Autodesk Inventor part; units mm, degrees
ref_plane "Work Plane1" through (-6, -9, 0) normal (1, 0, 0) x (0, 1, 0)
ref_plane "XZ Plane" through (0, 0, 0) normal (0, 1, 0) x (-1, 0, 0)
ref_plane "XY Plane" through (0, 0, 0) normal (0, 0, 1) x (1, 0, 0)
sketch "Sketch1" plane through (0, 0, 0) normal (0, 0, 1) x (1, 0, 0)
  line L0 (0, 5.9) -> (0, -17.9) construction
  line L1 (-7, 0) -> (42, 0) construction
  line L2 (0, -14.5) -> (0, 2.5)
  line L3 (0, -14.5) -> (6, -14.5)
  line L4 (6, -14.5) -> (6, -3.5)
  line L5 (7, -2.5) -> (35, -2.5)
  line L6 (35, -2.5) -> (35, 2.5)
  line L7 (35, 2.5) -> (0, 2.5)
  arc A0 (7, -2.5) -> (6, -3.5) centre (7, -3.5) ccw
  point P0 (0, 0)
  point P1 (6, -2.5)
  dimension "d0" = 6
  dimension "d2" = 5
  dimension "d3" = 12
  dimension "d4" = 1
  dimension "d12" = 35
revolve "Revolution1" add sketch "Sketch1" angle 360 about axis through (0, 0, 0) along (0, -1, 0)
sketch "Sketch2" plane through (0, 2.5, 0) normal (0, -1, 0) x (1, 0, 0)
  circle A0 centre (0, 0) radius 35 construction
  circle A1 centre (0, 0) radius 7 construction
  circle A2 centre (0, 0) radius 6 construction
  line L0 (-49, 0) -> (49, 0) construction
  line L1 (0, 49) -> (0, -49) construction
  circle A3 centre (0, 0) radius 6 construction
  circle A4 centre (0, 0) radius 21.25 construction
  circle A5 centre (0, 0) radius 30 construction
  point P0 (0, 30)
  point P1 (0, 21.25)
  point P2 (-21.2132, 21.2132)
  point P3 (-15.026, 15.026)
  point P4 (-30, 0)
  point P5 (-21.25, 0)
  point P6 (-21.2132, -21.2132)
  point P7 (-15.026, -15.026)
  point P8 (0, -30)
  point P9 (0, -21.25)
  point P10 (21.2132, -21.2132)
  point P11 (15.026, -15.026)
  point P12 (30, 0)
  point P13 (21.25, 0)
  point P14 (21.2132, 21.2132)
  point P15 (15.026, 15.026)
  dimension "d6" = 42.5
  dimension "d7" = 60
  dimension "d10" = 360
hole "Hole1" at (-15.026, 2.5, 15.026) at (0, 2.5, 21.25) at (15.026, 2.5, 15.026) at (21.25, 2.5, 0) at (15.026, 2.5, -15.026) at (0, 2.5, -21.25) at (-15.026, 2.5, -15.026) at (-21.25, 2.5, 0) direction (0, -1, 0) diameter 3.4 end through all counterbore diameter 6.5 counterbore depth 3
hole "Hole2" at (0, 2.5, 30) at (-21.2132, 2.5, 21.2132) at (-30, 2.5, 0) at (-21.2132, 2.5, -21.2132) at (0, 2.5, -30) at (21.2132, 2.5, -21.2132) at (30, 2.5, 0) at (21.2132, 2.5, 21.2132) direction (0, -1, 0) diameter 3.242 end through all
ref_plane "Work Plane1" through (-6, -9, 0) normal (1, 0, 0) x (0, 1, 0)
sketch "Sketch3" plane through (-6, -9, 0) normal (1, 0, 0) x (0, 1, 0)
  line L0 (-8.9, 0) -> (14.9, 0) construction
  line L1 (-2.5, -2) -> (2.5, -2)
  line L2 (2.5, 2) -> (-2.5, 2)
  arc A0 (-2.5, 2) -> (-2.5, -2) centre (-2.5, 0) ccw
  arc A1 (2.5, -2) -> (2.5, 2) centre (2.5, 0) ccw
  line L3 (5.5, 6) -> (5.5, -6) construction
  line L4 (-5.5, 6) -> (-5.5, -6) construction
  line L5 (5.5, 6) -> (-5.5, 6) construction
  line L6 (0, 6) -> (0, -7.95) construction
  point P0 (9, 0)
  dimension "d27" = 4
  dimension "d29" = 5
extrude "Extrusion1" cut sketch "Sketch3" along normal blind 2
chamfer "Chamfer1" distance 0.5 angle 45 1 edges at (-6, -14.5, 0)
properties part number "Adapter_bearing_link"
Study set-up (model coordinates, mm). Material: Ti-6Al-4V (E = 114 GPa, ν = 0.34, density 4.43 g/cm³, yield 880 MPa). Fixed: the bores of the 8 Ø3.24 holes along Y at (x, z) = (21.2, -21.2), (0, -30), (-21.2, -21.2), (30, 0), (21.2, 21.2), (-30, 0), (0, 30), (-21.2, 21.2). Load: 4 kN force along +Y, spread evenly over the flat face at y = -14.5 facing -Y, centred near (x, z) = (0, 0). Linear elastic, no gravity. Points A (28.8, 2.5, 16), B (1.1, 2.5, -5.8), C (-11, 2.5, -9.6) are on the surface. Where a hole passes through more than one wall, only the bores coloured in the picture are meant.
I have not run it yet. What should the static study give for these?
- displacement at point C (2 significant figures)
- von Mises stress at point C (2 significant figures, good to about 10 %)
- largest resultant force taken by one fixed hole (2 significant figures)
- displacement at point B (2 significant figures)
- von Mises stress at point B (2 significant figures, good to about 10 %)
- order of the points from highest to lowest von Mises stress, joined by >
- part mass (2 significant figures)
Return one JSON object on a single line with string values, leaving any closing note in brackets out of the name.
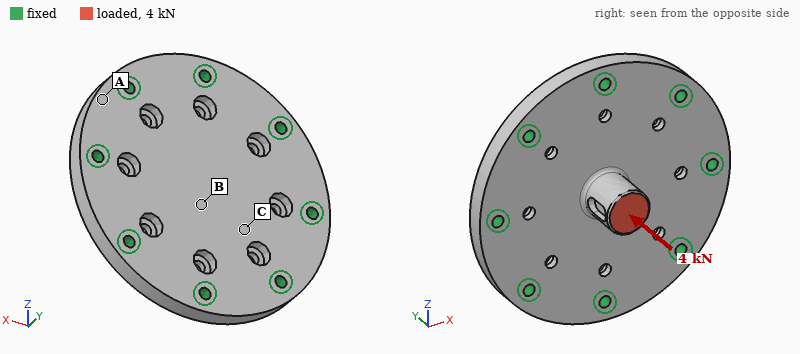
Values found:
{"displacement at point C": "32 µm", "von Mises stress at point C": "52 MPa", "largest resultant force taken by one fixed hole": "500 N", "displacement at point B": "50 µm", "von Mises stress at point B": "110 MPa", "order of the points from highest to lowest von Mises stress, joined by >": "B > C > A", "part mass": "85 g"}
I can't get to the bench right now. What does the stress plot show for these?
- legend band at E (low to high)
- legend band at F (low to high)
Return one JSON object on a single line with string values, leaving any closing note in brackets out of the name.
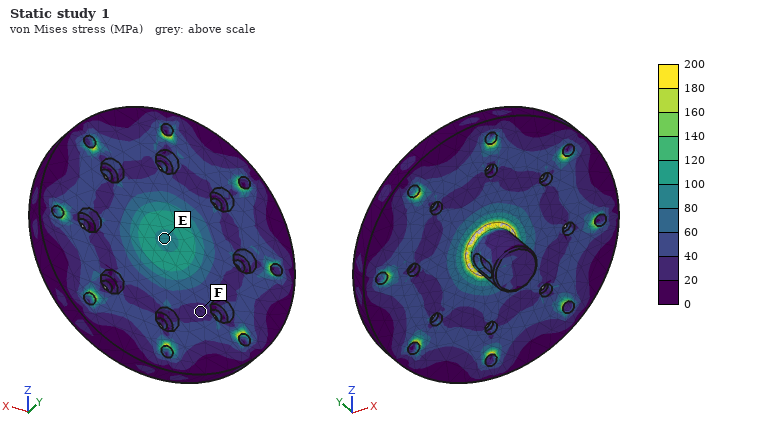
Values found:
{"legend band at E": "80 to 100 MPa", "legend band at F": "20 to 40 MPa"}
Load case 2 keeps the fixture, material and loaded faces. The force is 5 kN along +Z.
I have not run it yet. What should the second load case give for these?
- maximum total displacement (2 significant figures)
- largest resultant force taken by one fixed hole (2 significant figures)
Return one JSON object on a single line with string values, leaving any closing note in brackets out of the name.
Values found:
{"maximum total displacement": "0.13 mm", "largest resultant force taken by one fixed hole": "1.3 kN"}
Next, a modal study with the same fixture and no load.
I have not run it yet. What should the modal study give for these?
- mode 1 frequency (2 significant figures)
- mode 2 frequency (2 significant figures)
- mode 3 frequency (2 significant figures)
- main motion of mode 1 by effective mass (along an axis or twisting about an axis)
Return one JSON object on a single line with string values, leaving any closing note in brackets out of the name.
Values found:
{"mode 1 frequency": "9800 Hz", "mode 2 frequency": "17 kHz", "mode 3 frequency": "17 kHz", "main motion of mode 1 by effective mass": "along Y"}
